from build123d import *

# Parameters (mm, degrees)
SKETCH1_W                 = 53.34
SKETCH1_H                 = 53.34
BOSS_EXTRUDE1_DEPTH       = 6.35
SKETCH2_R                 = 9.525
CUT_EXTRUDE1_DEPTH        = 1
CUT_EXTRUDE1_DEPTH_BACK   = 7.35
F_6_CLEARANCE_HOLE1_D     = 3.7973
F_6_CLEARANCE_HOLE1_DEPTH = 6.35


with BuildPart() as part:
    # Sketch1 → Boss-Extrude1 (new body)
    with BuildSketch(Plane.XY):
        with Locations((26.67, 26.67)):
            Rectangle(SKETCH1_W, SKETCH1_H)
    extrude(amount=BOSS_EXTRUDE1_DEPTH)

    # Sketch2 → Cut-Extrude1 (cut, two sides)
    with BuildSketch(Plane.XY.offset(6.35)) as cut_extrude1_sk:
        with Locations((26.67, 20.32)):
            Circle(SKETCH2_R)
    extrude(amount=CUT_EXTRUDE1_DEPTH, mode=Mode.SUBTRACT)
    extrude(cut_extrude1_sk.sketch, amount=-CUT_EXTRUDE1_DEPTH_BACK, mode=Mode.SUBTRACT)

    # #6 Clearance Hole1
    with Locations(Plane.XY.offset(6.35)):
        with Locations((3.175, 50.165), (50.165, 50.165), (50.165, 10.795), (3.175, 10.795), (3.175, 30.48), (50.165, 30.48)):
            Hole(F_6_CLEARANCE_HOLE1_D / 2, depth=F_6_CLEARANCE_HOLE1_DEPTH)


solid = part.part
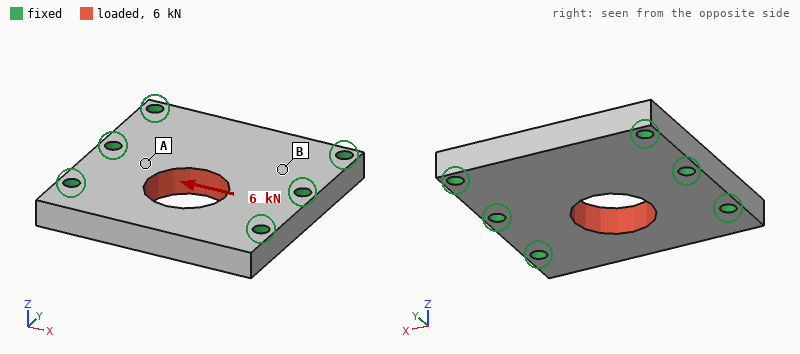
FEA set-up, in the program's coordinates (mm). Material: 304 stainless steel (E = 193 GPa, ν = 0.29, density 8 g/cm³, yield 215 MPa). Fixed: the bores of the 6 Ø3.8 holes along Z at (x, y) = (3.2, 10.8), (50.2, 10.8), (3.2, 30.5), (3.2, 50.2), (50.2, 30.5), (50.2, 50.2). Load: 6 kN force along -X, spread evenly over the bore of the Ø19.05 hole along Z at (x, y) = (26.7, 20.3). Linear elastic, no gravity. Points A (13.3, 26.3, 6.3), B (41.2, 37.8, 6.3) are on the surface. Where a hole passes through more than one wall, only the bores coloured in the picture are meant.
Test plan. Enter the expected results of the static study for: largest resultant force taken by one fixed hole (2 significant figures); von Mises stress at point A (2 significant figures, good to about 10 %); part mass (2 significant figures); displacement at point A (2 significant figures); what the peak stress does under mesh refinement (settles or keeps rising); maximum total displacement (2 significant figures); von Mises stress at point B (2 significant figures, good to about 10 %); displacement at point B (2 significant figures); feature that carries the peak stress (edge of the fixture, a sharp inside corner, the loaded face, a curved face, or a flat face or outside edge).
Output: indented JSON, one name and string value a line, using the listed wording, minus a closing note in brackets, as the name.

{
  "largest resultant force taken by one fixed hole": "1.5 kN",
  "von Mises stress at point A": "16 MPa",
  "part mass": "130 g",
  "displacement at point A": "0.97 µm",
  "what the peak stress does under mesh refinement": "keeps rising",
  "maximum total displacement": "2.1 µm",
  "von Mises stress at point B": "5.1 MPa",
  "displacement at point B": "0.48 µm",
  "feature that carries the peak stress": "edge of the fixture"
}
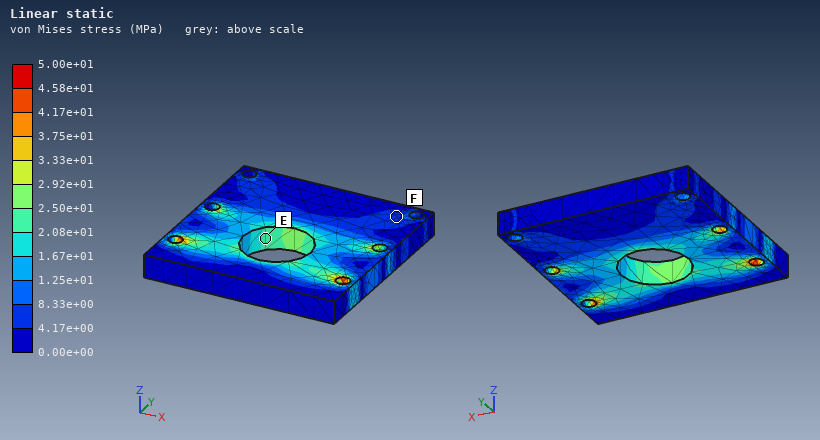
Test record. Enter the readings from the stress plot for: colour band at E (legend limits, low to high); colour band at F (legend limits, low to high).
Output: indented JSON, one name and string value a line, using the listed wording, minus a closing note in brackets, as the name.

{
  "colour band at E": "2.08e+01 to 2.50e+01 MPa",
  "colour band at F": "4.17e+00 to 8.33e+00 MPa"
}
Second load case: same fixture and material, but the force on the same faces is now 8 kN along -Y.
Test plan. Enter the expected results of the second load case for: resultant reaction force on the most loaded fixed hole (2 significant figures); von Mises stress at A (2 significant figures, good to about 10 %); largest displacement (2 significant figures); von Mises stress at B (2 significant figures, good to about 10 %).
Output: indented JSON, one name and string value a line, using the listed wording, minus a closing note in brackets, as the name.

{
  "resultant reaction force on the most loaded fixed hole": "1.8 kN",
  "von Mises stress at A": "29 MPa",
  "largest displacement": "6.3 µm",
  "von Mises stress at B": "20 MPa"
}
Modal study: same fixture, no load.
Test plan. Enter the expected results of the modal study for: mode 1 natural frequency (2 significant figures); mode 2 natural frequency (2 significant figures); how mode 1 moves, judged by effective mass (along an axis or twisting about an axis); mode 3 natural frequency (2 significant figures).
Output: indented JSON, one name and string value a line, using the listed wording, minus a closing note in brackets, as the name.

{
  "mode 1 natural frequency": "13 kHz",
  "mode 2 natural frequency": "14 kHz",
  "how mode 1 moves, judged by effective mass": "along Z",
  "mode 3 natural frequency": "22 kHz"
}
